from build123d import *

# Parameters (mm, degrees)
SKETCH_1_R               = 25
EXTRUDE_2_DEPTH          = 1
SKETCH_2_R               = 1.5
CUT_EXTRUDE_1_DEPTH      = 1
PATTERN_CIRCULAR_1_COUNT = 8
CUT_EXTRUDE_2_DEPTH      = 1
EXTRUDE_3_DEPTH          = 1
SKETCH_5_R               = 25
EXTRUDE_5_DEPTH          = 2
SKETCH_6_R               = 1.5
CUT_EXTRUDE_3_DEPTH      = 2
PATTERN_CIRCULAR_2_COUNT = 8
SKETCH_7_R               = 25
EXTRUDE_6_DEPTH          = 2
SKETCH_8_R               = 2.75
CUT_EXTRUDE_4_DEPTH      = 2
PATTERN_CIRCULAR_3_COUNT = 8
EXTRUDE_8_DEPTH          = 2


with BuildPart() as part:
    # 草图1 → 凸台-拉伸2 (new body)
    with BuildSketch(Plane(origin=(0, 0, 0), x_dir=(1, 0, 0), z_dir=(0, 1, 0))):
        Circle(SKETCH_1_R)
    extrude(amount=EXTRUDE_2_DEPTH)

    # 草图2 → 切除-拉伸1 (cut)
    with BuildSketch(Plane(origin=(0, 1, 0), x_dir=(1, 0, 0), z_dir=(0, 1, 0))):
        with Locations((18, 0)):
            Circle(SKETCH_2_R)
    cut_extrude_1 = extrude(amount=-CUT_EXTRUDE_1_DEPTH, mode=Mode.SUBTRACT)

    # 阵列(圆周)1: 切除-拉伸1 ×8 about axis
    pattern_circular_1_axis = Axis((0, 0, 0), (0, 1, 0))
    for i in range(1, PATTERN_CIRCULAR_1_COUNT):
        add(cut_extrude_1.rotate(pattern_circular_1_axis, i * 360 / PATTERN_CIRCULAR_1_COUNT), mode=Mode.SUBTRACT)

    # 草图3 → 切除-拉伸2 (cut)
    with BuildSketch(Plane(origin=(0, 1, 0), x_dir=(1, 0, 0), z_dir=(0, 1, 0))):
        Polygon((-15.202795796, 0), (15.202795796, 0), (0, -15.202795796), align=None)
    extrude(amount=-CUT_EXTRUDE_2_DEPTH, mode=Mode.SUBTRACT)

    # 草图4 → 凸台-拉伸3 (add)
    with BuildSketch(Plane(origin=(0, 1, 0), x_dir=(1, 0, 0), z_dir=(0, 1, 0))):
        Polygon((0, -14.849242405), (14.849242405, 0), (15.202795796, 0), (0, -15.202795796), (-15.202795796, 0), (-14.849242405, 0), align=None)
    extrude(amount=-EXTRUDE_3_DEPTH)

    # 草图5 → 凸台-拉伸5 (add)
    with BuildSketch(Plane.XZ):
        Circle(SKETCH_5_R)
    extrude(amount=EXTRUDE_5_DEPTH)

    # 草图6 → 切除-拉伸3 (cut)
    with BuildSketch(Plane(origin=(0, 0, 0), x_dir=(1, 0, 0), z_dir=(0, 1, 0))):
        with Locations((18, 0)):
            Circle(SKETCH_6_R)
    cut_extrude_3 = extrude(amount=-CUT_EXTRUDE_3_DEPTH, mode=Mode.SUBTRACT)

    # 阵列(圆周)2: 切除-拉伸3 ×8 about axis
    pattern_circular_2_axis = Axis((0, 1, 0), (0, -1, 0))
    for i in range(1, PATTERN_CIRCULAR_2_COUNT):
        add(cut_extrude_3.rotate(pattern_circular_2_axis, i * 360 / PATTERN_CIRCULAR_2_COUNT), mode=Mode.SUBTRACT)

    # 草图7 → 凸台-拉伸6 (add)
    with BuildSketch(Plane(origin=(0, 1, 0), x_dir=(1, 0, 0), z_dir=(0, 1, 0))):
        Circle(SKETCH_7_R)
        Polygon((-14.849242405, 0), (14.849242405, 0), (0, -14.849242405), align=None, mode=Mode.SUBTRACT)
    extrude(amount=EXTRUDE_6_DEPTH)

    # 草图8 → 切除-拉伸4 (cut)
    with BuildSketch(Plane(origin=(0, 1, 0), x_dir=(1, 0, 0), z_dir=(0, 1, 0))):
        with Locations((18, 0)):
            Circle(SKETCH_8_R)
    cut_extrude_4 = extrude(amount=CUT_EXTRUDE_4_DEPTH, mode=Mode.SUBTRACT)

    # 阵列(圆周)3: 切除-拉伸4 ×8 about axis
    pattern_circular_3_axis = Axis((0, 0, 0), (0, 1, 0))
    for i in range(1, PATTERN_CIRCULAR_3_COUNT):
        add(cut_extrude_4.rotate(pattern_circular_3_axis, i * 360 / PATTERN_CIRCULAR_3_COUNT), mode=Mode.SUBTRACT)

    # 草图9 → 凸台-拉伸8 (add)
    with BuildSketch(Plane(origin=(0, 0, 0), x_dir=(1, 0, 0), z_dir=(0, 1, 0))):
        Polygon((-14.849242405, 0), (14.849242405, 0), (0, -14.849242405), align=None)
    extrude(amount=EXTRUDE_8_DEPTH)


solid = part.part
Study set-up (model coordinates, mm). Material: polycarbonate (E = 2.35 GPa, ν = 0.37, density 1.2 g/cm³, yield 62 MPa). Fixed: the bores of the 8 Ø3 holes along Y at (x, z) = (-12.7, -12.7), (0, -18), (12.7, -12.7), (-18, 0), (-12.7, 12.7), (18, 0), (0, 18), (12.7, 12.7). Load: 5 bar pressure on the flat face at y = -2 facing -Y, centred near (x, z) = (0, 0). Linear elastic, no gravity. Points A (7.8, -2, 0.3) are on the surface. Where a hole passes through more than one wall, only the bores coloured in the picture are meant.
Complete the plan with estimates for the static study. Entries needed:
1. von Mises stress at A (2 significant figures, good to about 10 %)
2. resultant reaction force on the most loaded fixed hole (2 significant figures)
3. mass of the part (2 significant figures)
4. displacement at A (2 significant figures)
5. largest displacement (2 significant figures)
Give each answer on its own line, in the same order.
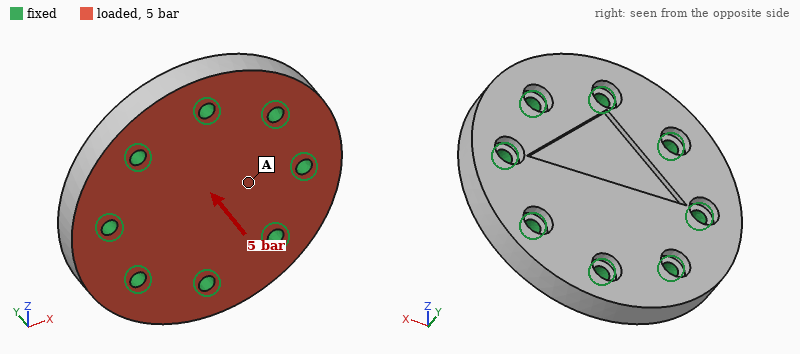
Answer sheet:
2.6 MPa
120 N
11 g
43 µm
58 µm
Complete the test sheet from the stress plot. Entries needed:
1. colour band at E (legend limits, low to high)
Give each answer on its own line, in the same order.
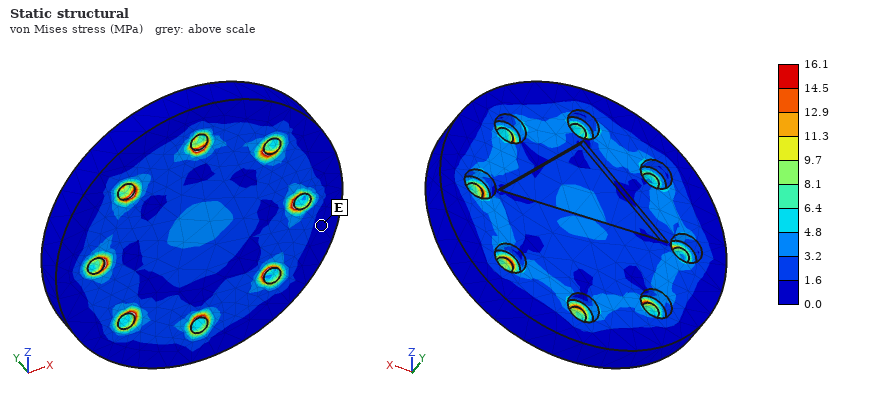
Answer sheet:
0.0 to 1.6 MPa
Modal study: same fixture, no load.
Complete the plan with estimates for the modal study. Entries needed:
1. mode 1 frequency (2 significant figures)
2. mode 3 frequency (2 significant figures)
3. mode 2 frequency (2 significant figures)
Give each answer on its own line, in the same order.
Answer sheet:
6900 Hz
11 kHz
11 kHz
